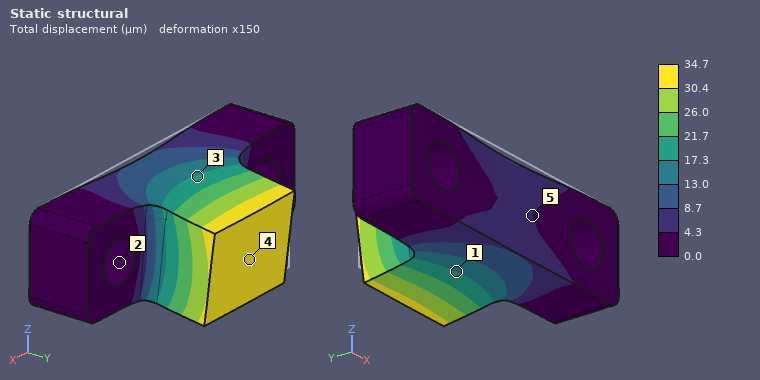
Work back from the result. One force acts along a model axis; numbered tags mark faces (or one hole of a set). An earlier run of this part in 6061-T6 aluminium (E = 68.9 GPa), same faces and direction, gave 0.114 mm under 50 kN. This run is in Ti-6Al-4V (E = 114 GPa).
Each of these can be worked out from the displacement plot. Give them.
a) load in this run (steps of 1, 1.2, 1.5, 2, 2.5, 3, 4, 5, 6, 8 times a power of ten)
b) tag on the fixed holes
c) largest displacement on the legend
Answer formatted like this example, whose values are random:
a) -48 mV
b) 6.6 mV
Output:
a) 25 kN
b) 2
c) 34.7 µm
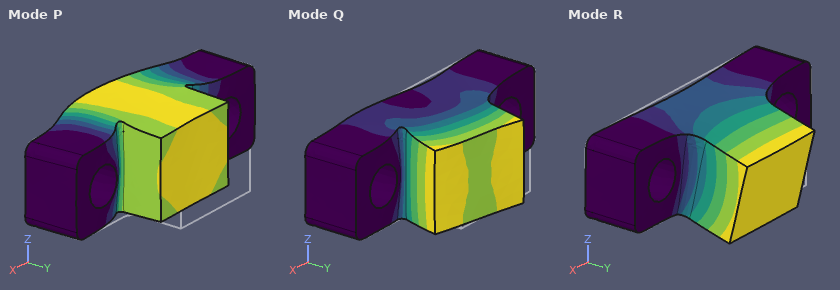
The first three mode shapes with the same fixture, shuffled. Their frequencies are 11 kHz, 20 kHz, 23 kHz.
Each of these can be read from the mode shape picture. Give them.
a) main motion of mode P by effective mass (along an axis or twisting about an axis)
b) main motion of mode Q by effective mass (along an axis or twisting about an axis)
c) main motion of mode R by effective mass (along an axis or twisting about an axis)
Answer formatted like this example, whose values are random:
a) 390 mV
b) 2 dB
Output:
a) along Y
b) along X
c) along Z
